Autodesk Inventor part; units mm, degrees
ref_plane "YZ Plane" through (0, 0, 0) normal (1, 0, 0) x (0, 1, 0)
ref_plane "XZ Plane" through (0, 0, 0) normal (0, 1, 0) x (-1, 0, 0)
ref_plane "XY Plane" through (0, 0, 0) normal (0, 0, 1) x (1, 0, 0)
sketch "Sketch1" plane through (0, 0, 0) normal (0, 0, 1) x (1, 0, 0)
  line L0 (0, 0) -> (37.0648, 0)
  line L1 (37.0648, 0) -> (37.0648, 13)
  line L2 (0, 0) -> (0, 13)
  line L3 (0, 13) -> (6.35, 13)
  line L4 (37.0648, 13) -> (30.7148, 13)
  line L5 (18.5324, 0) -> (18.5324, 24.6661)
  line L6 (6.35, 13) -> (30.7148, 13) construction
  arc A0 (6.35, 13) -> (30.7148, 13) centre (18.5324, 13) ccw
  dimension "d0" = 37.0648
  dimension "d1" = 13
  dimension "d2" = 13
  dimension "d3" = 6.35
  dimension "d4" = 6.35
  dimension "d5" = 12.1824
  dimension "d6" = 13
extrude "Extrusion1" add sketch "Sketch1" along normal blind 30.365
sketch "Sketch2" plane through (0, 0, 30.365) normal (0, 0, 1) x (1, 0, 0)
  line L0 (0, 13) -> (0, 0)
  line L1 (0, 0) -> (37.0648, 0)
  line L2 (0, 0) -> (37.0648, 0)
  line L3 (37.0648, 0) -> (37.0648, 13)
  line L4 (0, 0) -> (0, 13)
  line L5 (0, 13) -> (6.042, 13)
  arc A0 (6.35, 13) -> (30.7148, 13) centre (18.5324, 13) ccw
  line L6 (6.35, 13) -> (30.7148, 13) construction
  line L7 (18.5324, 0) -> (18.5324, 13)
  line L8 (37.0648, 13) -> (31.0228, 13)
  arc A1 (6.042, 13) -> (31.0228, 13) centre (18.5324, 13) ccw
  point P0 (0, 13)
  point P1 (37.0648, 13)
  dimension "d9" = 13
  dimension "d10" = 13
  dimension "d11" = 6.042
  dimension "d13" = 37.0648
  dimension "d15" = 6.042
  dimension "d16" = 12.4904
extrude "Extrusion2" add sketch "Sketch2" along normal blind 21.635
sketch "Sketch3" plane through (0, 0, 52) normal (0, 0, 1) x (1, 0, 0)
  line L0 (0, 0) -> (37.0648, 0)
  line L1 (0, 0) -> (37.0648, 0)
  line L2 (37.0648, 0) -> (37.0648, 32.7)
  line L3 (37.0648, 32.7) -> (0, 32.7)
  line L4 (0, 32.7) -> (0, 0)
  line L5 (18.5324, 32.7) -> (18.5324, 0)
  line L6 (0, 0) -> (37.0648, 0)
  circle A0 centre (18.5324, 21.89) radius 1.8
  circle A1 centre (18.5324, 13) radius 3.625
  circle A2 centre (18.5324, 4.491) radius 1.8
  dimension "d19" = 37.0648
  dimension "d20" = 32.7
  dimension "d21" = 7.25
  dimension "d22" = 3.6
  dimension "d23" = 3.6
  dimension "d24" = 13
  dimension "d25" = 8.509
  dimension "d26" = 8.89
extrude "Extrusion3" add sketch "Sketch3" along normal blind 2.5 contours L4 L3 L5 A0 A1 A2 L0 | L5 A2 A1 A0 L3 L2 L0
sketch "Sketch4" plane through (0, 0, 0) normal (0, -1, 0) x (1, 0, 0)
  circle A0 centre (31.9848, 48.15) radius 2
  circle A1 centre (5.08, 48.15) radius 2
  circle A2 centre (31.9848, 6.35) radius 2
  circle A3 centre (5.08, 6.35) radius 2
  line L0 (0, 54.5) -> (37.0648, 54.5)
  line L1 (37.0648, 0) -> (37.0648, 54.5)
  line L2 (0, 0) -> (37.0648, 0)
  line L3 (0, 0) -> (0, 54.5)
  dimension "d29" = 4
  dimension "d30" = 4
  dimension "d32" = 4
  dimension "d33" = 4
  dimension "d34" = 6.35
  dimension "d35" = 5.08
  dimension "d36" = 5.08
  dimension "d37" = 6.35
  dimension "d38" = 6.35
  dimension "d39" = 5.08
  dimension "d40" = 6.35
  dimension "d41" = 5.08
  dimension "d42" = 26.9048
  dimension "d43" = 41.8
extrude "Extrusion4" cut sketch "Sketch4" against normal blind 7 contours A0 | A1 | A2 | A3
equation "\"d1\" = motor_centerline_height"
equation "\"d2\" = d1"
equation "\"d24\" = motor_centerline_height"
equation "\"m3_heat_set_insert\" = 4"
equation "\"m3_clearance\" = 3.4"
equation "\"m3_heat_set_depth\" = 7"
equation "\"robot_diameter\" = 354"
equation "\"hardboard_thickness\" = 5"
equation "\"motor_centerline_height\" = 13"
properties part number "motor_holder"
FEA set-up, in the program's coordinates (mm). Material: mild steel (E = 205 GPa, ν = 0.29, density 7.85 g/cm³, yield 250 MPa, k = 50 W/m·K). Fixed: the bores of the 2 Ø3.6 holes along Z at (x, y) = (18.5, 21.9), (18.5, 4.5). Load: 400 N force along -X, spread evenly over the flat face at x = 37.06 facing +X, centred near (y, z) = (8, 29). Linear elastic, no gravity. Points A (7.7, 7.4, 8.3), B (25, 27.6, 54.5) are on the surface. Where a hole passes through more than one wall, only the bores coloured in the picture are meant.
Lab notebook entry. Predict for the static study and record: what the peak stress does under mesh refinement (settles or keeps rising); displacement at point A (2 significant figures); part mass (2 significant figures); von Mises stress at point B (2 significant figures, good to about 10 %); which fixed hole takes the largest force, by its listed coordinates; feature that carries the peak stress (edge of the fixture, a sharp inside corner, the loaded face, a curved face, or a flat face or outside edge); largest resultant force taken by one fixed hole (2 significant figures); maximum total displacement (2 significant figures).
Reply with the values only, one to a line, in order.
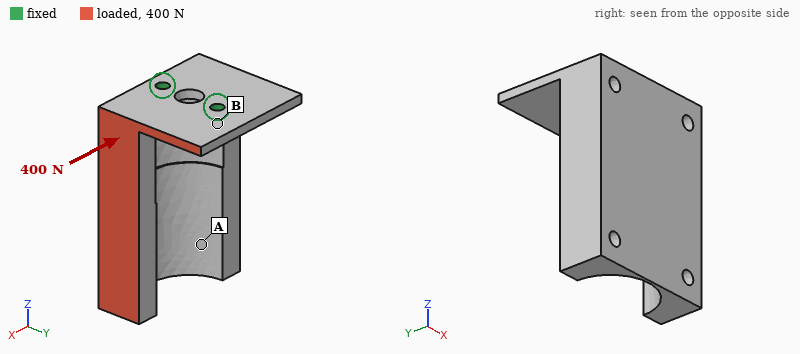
keeps rising
0.12 mm
120 g
44 MPa
(18.5, 4.5)
edge of the fixture
290 N
0.16 mm
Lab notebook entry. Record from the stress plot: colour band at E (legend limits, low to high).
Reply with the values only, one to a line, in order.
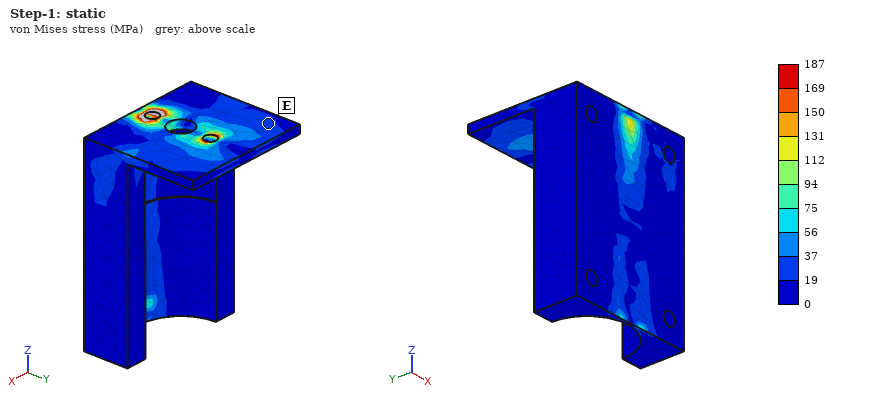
19 to 37 MPa
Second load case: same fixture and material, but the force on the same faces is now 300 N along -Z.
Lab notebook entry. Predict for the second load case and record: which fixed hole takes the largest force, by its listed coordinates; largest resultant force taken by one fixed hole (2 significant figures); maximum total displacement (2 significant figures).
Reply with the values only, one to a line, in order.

(18.5, 4.5)
230 N
81 µm
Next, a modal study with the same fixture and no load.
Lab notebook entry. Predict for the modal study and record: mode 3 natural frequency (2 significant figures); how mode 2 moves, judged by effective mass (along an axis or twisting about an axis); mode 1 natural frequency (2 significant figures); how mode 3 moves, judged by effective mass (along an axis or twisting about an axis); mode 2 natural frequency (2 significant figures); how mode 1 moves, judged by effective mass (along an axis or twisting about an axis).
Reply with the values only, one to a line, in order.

2900 Hz
along Y
910 Hz
twisting about Z
1100 Hz
along X
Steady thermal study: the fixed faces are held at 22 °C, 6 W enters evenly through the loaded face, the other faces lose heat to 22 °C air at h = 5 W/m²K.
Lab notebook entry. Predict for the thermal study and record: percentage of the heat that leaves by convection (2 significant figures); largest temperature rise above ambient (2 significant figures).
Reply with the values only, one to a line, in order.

9.9 %
29 K
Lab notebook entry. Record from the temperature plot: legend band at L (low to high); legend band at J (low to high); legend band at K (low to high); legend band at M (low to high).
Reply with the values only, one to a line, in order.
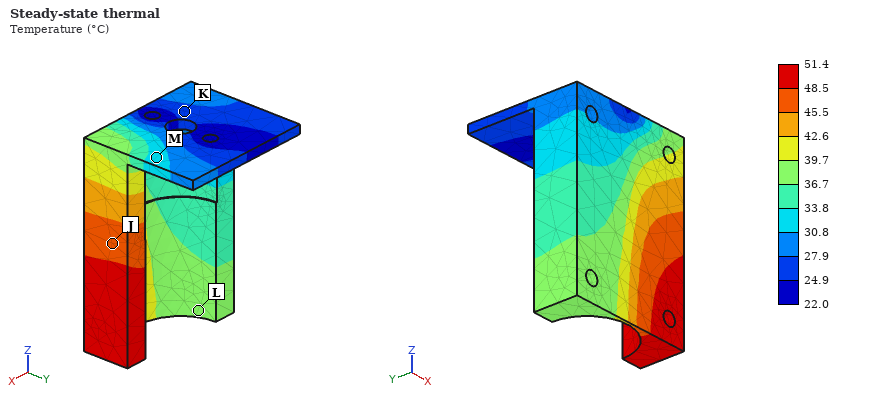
36.7 to 39.7 °C
45.5 to 48.5 °C
24.9 to 27.9 °C
30.8 to 33.8 °C
